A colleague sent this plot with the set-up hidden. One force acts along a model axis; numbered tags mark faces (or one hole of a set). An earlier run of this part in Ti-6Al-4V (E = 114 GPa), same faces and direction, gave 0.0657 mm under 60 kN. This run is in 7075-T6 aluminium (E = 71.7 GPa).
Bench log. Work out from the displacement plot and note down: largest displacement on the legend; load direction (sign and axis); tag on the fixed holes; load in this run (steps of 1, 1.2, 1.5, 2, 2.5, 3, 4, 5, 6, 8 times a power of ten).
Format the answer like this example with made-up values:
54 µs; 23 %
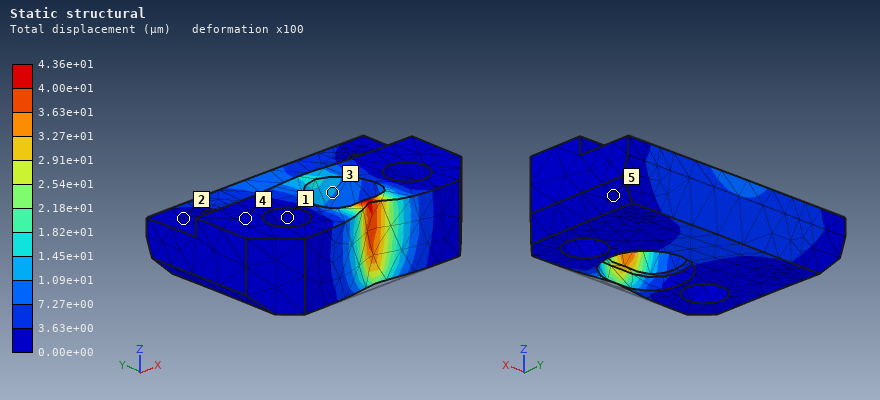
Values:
4.36e+01 µm; +Y; 1; 25 kN
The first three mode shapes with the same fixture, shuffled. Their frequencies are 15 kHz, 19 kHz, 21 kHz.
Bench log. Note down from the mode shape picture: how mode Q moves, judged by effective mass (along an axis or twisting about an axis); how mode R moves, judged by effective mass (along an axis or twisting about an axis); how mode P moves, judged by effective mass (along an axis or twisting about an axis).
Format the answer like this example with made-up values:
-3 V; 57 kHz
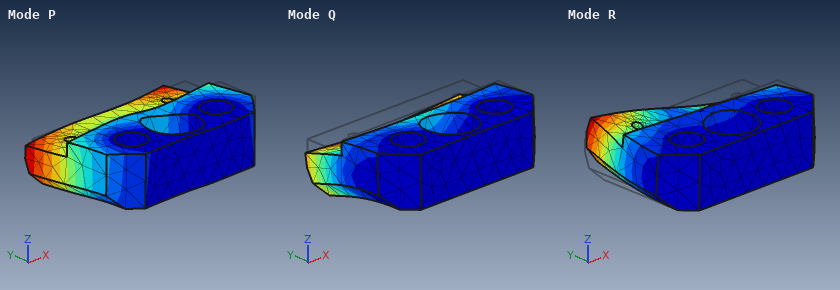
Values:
along Z; twisting about Y; along X
